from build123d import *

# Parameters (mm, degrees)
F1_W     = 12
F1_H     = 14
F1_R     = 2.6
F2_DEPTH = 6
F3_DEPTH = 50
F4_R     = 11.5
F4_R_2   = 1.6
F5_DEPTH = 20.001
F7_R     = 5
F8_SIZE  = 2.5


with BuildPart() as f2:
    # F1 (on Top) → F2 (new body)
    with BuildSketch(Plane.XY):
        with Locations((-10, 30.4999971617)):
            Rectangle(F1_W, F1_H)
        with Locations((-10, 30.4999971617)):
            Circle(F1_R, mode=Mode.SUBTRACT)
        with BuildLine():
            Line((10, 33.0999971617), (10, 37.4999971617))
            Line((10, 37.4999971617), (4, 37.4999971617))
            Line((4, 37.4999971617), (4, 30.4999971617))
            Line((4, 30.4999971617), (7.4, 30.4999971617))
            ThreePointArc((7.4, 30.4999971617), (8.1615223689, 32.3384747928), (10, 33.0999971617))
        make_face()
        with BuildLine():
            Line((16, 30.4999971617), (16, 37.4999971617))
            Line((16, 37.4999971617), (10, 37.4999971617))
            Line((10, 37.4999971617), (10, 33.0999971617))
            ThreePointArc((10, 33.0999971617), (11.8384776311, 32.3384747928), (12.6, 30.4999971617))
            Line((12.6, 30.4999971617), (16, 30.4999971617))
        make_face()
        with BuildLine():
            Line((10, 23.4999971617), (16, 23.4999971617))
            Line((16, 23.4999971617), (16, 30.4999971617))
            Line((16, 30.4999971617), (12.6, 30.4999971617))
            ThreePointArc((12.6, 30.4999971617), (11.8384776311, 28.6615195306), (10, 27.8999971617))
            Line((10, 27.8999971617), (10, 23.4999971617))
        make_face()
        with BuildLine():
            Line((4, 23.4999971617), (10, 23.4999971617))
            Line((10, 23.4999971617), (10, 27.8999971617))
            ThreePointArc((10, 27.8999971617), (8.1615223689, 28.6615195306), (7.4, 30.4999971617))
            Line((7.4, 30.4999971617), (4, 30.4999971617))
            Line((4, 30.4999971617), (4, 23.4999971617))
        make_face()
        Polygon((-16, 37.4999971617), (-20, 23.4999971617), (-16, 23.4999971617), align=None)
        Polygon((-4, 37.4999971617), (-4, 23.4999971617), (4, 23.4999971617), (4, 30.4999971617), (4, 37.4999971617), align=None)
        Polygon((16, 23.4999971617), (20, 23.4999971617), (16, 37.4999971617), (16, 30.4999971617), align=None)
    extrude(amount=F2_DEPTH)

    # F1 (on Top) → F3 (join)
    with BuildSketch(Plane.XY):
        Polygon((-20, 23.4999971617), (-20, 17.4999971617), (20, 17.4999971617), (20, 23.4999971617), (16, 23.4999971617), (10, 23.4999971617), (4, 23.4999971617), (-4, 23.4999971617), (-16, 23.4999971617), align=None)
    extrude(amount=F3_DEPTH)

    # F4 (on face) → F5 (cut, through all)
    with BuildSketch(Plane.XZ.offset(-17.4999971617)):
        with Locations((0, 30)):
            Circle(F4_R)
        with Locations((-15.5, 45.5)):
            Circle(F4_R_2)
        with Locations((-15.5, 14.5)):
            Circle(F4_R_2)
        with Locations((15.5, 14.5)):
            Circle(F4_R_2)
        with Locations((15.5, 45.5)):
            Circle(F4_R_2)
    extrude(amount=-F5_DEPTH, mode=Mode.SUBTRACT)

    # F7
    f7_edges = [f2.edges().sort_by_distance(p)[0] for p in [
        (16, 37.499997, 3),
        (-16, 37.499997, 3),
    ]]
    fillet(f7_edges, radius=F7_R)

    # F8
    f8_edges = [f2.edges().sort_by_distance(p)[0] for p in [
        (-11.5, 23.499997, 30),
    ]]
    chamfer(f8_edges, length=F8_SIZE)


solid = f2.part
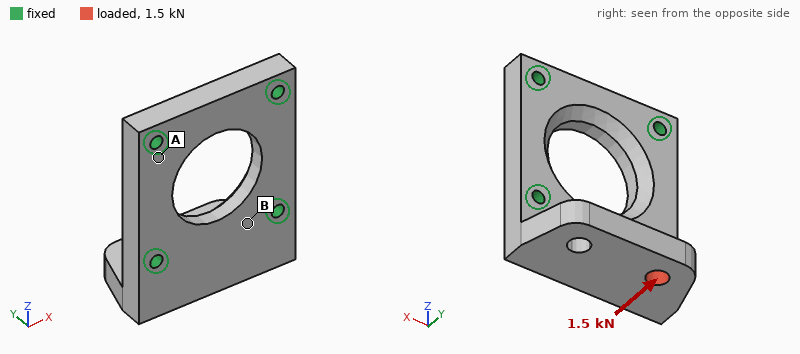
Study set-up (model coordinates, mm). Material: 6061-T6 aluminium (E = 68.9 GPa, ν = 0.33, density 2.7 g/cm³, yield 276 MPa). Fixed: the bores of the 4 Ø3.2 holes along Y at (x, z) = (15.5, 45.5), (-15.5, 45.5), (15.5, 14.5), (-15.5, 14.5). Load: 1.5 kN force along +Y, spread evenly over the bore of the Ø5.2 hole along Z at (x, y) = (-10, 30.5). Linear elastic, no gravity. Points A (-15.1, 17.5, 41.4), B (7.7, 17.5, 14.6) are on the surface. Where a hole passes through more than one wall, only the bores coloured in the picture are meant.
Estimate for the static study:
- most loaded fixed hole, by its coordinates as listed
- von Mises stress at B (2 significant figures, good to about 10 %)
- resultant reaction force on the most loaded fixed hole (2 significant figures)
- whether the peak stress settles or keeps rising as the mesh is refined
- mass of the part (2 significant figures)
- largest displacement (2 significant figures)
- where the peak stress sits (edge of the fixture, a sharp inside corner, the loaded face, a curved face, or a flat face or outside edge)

(-15.5, 14.5)
29 MPa
1.3 kN
keeps rising
32 g
75 µm
edge of the fixture
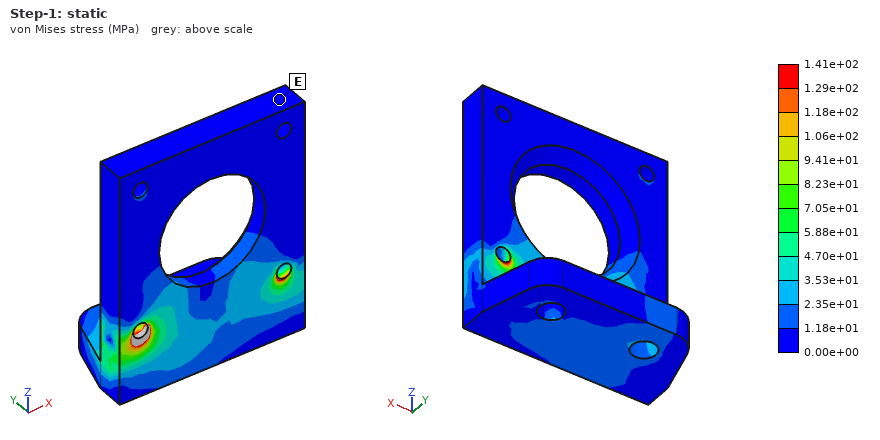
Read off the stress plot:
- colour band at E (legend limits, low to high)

0.00e+00 to 1.18e+01 MPa
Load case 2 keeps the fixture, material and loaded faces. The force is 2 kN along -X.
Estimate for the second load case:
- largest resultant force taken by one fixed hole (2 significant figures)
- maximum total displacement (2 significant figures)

1.4 kN
29 µm
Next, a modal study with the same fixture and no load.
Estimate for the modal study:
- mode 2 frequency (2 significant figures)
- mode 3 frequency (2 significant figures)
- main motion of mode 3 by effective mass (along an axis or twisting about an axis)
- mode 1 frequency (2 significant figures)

14 kHz
18 kHz
along Y
7500 Hz
